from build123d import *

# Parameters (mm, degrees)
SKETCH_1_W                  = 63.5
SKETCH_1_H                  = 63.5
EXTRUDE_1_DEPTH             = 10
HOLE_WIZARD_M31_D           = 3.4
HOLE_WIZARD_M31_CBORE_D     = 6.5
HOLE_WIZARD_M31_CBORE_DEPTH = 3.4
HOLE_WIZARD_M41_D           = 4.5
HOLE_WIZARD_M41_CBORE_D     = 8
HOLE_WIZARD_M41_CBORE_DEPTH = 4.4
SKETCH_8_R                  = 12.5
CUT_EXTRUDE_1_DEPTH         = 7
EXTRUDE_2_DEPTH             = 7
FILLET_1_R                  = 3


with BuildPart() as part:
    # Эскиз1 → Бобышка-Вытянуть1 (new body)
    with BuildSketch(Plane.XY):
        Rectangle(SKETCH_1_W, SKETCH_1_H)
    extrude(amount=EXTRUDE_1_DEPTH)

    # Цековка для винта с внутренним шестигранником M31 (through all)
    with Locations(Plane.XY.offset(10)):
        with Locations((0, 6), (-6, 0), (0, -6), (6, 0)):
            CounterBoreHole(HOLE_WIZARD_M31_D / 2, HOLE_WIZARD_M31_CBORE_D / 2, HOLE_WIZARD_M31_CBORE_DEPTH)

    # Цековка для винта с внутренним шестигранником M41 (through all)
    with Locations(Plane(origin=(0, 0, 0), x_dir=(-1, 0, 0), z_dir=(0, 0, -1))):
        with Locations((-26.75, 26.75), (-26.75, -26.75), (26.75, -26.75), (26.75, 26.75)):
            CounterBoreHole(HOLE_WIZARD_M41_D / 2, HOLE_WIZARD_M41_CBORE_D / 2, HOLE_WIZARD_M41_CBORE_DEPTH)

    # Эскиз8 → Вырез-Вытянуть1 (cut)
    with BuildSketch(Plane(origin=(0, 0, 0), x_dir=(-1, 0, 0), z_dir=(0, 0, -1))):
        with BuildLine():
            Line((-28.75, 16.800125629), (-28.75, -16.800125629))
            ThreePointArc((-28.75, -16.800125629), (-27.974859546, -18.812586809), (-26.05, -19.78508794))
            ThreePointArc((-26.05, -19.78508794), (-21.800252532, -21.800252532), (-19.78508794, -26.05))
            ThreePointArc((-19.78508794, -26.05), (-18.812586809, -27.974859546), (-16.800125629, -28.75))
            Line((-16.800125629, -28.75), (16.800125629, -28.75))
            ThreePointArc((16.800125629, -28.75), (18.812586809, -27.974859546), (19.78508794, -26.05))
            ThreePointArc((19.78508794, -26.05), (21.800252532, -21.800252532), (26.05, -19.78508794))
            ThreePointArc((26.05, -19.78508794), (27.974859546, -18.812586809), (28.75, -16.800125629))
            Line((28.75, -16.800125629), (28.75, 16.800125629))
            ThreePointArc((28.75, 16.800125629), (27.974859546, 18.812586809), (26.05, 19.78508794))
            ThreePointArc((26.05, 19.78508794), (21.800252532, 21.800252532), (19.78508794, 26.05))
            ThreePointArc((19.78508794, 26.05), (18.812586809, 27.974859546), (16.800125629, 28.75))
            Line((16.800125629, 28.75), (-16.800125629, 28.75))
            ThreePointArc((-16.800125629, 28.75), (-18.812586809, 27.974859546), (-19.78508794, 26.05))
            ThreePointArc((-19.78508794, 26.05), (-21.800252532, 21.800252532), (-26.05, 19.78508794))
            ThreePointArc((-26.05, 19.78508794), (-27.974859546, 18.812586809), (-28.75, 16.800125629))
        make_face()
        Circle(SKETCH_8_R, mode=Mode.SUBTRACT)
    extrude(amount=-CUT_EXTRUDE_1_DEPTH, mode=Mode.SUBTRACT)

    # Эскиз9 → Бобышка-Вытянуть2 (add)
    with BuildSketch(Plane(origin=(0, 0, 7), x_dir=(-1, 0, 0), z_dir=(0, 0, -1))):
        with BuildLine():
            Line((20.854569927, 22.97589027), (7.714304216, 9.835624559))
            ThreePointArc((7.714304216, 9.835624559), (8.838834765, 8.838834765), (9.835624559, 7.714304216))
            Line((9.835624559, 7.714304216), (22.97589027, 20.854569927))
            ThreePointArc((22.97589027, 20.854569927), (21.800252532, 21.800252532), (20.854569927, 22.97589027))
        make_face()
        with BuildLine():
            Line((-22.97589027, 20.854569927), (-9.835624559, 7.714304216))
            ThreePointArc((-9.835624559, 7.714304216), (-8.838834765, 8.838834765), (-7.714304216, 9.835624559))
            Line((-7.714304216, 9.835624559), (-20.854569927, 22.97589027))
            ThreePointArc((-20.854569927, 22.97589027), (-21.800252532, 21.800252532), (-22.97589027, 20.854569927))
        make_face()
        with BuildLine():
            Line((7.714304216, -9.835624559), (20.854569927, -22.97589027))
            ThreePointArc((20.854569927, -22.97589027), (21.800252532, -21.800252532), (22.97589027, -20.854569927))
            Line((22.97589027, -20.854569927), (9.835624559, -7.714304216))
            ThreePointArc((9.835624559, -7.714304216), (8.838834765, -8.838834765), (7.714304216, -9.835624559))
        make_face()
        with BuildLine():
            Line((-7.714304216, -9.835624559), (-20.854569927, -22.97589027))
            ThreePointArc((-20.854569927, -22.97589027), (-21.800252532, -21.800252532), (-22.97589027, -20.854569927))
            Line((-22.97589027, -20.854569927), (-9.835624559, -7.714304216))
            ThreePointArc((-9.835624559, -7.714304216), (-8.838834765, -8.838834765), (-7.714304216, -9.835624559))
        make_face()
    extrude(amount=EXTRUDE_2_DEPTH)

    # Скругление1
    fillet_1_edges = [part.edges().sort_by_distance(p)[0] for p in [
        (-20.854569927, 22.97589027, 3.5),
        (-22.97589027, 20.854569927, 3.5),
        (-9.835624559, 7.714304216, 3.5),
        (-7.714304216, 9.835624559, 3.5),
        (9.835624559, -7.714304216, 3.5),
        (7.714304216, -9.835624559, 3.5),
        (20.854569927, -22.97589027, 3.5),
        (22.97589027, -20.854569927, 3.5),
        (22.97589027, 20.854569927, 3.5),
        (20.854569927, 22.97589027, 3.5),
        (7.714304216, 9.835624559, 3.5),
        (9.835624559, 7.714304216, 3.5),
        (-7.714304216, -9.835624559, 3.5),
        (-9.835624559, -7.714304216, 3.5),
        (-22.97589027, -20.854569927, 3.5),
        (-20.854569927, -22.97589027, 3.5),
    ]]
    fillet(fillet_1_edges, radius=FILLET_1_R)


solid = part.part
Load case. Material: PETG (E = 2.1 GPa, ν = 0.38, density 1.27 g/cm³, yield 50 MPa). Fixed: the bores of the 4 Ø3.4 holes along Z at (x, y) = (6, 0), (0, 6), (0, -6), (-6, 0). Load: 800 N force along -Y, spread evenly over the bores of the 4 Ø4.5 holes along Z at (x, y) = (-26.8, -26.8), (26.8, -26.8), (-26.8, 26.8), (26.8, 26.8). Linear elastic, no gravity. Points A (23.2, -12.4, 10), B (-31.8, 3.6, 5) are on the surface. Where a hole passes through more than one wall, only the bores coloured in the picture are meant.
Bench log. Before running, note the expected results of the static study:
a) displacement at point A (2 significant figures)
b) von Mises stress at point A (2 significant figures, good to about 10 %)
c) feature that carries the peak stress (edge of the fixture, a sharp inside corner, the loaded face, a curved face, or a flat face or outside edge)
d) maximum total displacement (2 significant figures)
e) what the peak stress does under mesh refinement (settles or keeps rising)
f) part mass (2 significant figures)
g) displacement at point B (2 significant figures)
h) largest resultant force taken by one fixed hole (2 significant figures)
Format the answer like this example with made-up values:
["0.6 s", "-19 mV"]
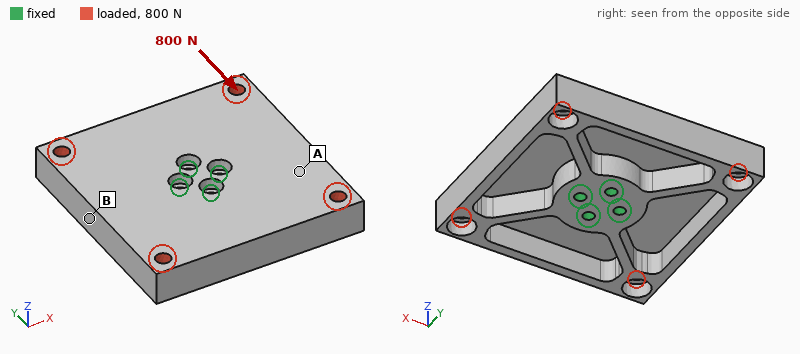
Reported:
["0.077 mm", "2.7 MPa", "edge of the fixture", "0.14 mm", "keeps rising", "28 g", "0.077 mm", "280 N"]
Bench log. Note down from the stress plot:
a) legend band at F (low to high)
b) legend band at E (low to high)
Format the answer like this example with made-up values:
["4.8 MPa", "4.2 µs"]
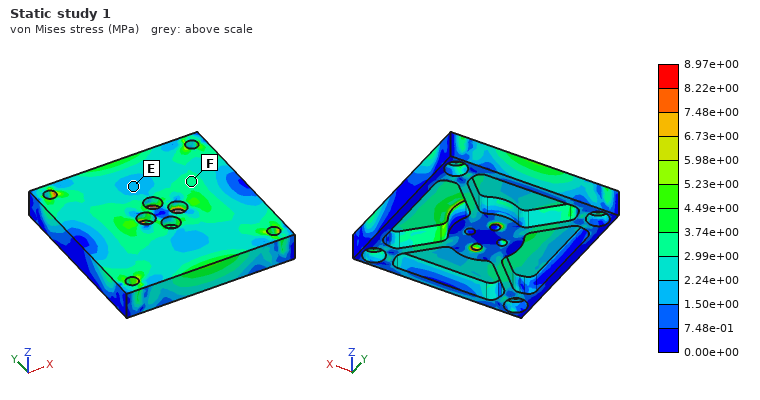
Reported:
["2.99e+00 to 3.74e+00 MPa", "1.50e+00 to 2.24e+00 MPa"]
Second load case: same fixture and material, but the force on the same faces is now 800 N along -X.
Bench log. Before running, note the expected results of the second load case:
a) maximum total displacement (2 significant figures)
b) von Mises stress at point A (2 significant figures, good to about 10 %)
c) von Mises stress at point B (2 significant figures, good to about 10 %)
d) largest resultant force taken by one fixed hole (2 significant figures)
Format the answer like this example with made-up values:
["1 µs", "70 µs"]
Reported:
["0.14 mm", "2.6 MPa", "3.4 MPa", "280 N"]
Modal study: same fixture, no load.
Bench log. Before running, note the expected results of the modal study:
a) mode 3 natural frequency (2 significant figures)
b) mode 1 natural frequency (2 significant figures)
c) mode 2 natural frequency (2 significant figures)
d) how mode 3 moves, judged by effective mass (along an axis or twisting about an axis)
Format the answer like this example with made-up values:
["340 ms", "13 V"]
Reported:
["1300 Hz", "1000 Hz", "1000 Hz", "along Z"]
